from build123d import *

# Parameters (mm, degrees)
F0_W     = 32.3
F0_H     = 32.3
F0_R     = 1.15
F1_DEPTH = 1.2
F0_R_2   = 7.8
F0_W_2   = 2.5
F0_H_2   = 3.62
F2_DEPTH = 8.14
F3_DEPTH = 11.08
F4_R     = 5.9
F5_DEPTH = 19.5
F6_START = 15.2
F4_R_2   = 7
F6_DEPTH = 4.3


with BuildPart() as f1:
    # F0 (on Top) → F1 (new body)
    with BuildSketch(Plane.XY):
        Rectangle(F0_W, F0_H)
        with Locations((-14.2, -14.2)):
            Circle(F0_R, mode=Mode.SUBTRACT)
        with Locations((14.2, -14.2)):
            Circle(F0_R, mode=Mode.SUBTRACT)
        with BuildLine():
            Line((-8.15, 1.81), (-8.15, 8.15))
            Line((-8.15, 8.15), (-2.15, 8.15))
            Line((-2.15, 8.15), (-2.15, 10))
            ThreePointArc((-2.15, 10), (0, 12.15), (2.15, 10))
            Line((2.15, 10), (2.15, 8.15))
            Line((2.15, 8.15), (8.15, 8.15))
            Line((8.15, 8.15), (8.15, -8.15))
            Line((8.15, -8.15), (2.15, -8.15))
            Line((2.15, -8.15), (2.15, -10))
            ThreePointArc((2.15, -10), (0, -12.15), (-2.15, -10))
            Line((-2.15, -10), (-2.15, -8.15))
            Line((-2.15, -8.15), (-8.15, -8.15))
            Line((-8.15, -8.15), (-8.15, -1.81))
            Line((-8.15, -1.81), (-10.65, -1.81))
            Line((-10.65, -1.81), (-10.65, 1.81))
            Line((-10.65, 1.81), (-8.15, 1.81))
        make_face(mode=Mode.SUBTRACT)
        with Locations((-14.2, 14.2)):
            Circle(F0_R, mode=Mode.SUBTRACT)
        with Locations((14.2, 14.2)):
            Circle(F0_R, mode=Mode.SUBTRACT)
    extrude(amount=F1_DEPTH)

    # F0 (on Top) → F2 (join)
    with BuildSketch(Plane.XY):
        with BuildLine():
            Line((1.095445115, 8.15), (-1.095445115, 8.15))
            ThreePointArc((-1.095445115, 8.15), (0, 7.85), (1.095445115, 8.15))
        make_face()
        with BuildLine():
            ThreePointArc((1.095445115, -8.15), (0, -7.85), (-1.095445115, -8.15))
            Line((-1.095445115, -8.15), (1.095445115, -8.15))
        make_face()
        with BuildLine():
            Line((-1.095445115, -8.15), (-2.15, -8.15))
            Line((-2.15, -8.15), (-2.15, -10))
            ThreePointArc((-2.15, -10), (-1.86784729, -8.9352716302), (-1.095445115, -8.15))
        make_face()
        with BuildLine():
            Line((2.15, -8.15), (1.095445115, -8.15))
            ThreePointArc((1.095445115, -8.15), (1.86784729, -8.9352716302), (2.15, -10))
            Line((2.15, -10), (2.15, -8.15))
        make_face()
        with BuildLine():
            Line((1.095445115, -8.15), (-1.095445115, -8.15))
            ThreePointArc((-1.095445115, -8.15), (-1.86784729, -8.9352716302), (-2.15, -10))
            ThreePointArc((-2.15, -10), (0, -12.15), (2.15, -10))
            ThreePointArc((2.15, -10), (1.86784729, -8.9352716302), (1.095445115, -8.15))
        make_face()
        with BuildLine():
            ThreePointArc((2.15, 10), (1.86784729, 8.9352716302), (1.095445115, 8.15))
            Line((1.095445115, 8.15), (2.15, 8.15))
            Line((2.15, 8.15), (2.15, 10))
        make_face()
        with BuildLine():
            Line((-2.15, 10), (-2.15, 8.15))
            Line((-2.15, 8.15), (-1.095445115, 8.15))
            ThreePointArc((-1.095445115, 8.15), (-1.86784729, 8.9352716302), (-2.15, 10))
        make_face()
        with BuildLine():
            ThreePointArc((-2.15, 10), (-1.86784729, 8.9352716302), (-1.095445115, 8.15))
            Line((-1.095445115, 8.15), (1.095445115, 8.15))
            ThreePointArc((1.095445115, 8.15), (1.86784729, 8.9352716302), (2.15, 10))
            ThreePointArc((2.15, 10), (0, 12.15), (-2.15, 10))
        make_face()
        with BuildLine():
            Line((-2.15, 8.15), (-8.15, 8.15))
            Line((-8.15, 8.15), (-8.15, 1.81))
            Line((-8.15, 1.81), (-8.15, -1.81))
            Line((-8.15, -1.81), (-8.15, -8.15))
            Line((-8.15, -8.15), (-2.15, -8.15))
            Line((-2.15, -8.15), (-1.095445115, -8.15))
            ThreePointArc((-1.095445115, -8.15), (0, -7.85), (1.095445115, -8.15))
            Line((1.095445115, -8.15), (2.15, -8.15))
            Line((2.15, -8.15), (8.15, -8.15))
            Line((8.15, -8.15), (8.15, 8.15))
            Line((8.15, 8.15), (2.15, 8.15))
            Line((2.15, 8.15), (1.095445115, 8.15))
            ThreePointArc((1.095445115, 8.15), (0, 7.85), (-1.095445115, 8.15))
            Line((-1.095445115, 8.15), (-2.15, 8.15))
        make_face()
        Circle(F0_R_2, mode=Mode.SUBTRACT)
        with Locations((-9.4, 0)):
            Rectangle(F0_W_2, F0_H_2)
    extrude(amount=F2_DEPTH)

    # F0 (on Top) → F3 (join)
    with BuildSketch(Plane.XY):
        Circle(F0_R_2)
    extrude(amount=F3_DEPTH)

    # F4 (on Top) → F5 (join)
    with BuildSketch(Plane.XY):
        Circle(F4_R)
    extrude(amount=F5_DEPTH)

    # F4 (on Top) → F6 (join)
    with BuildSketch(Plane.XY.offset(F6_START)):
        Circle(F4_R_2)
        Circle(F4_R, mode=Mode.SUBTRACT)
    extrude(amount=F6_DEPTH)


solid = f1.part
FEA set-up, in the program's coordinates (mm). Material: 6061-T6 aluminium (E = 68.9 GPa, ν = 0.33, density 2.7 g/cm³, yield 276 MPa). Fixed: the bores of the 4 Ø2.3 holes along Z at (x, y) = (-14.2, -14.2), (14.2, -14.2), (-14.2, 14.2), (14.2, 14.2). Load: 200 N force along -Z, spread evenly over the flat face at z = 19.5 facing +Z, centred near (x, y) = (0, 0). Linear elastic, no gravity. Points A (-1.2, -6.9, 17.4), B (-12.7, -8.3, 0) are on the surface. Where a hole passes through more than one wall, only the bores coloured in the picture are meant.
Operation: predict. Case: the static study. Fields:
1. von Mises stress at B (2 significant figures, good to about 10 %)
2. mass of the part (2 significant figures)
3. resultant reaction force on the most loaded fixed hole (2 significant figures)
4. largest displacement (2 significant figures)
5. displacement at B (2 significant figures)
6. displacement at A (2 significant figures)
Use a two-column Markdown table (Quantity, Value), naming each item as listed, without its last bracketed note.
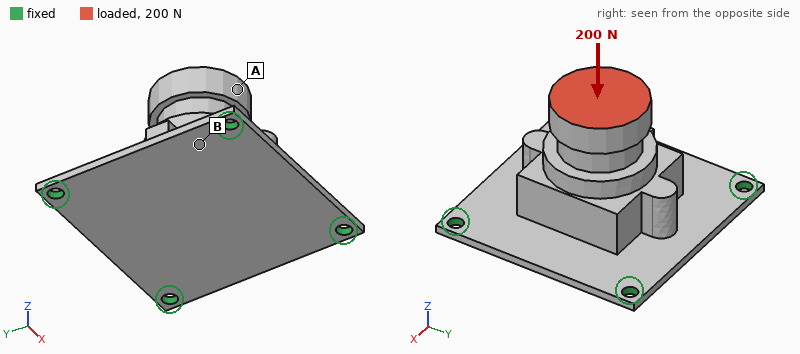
| Quantity | Value |
|---|---|
| von Mises stress at B | 18 MPa |
| mass of the part | 14 g |
| resultant reaction force on the most loaded fixed hole | 54 N |
| largest displacement | 37 µm |
| displacement at B | 19 µm |
| displacement at A | 36 µm |
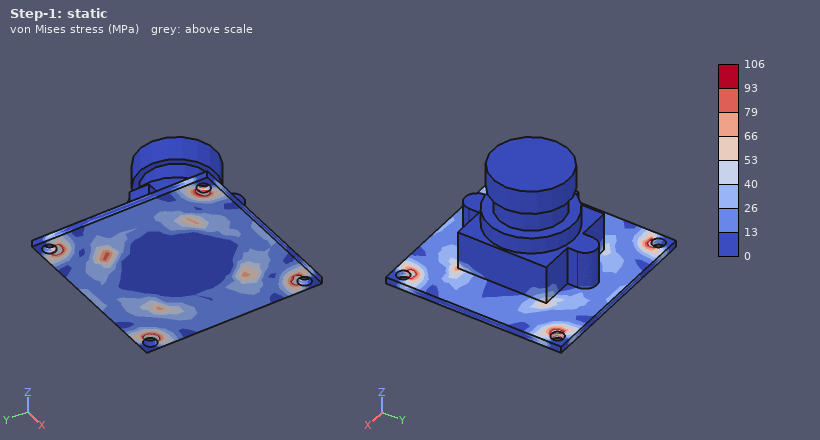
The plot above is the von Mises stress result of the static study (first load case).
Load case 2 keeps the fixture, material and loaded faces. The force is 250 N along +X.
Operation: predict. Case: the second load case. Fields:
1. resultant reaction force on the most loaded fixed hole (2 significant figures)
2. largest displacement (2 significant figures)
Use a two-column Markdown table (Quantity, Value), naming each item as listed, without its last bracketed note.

| Quantity | Value |
|---|---|
| resultant reaction force on the most loaded fixed hole | 120 N |
| largest displacement | 0.14 mm |
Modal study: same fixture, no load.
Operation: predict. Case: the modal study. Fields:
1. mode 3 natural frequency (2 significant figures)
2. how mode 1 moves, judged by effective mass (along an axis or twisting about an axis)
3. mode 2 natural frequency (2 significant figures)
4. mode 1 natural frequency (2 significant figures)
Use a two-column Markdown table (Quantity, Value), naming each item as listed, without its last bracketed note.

| Quantity | Value |
|---|---|
| mode 3 natural frequency | 3800 Hz |
| how mode 1 moves, judged by effective mass | along Z |
| mode 2 natural frequency | 3800 Hz |
| mode 1 natural frequency | 3400 Hz |
